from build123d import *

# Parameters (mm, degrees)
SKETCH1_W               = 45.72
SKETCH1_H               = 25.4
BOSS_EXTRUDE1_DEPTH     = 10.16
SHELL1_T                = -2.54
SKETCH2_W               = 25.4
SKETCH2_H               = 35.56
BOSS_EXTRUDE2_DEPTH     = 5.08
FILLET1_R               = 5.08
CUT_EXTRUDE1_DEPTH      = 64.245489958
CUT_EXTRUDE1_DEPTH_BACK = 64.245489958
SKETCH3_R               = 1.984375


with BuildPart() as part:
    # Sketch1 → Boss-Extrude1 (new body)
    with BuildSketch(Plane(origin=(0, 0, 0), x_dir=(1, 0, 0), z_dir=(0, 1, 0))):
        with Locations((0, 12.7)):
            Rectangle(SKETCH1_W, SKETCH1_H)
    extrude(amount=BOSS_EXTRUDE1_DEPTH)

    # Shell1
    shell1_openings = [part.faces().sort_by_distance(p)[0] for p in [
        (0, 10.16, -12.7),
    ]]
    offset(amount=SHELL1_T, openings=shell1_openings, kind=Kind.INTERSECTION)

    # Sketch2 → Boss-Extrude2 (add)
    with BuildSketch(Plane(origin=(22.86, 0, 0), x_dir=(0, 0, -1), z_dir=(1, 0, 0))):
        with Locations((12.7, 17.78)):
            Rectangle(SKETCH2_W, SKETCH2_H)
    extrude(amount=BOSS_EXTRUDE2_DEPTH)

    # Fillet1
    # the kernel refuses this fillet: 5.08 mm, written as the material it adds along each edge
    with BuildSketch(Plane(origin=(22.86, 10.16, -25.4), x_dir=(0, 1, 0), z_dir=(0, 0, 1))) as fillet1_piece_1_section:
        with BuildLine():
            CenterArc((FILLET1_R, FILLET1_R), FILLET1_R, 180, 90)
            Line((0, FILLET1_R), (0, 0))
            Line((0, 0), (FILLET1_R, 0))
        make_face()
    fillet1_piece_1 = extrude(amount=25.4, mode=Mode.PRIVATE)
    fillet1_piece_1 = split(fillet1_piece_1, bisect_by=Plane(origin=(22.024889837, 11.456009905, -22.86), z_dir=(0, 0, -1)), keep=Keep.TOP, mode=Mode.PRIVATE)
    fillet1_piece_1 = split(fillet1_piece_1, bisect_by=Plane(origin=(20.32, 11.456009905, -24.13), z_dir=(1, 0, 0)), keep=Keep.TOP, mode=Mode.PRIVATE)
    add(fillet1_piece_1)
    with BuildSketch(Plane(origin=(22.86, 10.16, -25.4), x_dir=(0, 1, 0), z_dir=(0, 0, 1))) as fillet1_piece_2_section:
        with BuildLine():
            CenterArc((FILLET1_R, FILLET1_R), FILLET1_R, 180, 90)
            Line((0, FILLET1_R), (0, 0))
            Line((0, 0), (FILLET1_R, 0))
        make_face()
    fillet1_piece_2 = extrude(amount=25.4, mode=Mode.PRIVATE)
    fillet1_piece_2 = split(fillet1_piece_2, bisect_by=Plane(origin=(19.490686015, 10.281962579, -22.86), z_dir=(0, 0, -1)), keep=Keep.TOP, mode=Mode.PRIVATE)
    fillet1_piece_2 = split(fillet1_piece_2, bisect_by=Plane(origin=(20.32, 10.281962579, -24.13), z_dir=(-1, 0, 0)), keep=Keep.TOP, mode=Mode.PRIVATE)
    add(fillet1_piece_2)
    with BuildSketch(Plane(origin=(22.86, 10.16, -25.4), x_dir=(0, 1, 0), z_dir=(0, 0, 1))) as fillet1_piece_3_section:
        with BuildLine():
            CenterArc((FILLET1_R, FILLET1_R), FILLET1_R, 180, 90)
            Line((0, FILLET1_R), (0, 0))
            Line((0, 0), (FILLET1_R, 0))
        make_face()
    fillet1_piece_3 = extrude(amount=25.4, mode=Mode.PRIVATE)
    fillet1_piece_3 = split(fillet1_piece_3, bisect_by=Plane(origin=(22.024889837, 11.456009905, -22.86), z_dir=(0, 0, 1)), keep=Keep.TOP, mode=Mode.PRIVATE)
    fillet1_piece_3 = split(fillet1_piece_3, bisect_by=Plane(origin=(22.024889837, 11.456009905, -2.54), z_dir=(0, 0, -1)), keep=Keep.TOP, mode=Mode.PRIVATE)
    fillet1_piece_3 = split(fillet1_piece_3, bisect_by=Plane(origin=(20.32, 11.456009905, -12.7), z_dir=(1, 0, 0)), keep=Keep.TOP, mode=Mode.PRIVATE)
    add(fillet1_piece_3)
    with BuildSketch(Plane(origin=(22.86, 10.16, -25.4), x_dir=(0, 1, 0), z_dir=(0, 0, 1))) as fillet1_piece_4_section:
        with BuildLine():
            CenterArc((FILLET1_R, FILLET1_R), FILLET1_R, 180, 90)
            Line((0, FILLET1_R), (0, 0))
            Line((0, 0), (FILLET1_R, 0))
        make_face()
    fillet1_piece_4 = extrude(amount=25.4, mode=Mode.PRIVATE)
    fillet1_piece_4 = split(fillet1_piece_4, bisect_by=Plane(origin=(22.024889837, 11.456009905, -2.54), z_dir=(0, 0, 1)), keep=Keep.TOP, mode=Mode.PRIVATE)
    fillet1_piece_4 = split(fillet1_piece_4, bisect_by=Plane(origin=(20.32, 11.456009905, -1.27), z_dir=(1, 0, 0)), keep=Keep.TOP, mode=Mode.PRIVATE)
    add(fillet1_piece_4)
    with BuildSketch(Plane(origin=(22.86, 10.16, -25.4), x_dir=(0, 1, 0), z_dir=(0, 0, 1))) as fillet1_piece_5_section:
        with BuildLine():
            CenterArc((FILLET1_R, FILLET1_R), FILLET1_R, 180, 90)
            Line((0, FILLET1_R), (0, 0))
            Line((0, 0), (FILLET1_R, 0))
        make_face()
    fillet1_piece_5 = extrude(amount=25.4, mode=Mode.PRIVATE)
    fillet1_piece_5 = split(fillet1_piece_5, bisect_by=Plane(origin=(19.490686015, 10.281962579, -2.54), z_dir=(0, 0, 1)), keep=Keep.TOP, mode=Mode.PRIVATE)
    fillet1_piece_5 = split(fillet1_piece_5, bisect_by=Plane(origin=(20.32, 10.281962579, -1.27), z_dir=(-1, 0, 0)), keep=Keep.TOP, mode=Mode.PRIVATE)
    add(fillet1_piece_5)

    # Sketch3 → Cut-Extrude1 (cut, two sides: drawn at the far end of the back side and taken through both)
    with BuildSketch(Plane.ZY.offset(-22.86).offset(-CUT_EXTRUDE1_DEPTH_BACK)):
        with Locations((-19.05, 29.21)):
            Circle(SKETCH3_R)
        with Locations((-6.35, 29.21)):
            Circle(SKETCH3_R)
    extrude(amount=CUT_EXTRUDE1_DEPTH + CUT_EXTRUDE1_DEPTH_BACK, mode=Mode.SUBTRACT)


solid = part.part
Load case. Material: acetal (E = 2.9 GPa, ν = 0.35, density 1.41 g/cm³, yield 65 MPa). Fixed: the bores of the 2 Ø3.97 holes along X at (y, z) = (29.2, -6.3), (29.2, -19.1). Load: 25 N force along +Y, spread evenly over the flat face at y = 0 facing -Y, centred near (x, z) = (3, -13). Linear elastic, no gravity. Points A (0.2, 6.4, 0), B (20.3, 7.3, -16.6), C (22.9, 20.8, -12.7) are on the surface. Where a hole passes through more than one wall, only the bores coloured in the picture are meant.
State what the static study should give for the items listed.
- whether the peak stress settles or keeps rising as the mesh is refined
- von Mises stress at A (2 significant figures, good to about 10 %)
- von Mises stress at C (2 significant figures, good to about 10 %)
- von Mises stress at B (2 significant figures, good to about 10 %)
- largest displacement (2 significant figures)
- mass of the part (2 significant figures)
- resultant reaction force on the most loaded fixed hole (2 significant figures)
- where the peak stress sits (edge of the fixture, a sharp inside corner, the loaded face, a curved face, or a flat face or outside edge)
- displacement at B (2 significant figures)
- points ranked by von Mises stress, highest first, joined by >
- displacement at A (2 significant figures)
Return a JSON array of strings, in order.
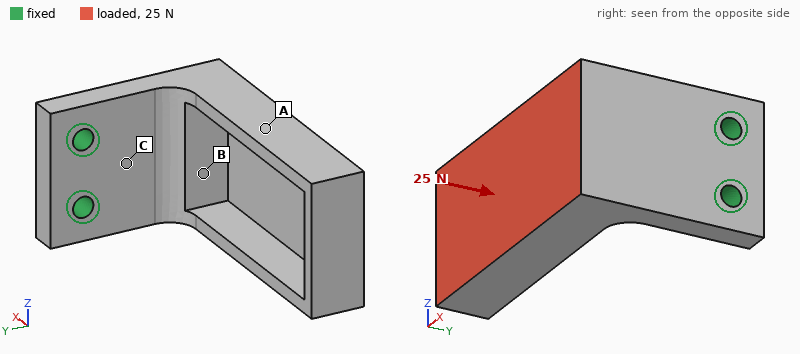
["keeps rising", "0.74 MPa", "4.9 MPa", "1.9 MPa", "0.79 mm", "14 g", "13 N", "edge of the fixture", "0.17 mm", "C > B > A", "0.40 mm"]
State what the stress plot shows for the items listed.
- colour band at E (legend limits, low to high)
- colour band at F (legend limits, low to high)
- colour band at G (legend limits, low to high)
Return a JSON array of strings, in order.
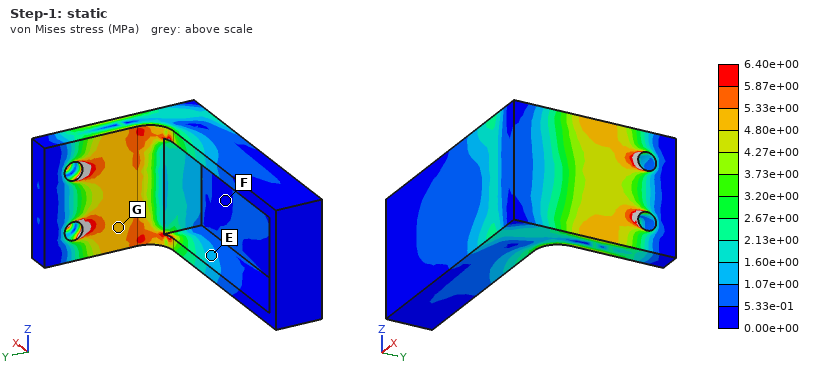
["1.07e+00 to 1.60e+00 MPa", "0.00e+00 to 5.33e-01 MPa", "4.80e+00 to 5.33e+00 MPa"]
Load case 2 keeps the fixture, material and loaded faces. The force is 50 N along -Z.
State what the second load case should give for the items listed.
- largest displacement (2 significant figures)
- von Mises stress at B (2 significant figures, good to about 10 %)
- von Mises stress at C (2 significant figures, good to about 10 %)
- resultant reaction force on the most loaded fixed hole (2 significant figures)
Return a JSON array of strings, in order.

["0.77 mm", "4.7 MPa", "7.2 MPa", "120 N"]
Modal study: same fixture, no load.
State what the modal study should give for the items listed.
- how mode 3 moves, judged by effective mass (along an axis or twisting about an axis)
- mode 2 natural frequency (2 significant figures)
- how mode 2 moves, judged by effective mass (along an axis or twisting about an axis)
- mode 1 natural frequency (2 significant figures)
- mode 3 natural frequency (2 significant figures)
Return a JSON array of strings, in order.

["along X", "490 Hz", "along Z", "330 Hz", "1300 Hz"]
